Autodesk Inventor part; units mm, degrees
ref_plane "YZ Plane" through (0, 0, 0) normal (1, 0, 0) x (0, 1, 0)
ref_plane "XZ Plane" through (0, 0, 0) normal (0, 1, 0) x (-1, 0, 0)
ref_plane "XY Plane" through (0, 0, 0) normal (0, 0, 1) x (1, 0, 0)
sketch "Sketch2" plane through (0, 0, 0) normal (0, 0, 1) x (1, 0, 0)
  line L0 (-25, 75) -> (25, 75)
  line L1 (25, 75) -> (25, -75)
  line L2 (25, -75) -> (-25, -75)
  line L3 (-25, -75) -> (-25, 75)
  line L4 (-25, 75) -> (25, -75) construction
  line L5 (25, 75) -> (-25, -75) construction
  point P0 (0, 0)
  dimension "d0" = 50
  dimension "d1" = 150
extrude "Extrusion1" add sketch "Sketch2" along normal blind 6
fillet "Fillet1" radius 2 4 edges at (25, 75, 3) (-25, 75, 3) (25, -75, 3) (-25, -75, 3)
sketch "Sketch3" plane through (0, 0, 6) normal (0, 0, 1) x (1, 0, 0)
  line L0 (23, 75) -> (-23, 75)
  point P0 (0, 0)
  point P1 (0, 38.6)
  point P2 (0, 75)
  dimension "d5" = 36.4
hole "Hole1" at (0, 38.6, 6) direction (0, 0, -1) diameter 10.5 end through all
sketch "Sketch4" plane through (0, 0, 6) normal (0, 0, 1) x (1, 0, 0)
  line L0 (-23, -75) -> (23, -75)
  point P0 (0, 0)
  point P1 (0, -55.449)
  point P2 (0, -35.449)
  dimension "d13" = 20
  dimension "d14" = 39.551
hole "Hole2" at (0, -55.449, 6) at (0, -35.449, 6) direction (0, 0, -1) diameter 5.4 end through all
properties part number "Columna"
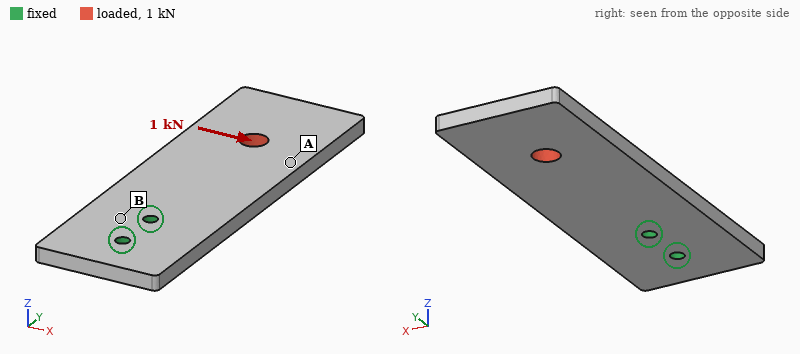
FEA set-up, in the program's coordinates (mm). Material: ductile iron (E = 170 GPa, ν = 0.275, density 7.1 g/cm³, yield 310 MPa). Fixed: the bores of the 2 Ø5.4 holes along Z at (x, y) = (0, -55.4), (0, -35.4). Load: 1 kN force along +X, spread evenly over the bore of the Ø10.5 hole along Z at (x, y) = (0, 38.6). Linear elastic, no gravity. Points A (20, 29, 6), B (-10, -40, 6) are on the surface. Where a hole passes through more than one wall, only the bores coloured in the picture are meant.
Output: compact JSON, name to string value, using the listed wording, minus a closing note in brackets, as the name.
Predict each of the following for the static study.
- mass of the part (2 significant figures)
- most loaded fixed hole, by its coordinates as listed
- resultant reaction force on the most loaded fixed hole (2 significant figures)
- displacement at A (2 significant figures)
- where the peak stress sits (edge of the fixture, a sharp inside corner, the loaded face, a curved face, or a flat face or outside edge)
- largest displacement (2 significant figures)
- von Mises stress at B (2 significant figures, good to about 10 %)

{"mass of the part": "310 g", "most loaded fixed hole, by its coordinates as listed": "(0, -35.4)", "resultant reaction force on the most loaded fixed hole": "3.9 kN", "displacement at A": "35 µm", "where the peak stress sits": "edge of the fixture", "largest displacement": "60 µm", "von Mises stress at B": "27 MPa"}
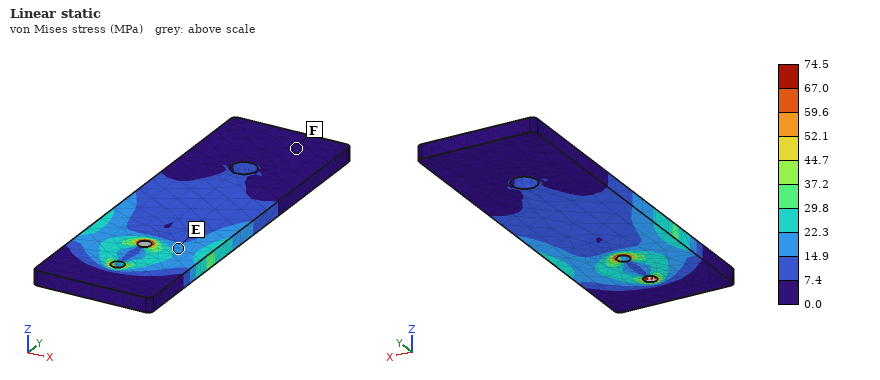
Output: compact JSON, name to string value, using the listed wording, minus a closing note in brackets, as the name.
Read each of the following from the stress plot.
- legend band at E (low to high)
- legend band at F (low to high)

{"legend band at E": "14.9 to 22.3 MPa", "legend band at F": "0.0 to 7.4 MPa"}
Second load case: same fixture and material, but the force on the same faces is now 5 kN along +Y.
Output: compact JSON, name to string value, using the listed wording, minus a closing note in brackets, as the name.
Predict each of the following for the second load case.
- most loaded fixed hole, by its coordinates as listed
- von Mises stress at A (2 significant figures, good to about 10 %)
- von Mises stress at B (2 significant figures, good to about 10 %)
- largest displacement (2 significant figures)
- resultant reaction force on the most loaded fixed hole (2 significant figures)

{"most loaded fixed hole, by its coordinates as listed": "(0, -35.4)", "von Mises stress at A": "11 MPa", "von Mises stress at B": "14 MPa", "largest displacement": "11 µm", "resultant reaction force on the most loaded fixed hole": "3.5 kN"}
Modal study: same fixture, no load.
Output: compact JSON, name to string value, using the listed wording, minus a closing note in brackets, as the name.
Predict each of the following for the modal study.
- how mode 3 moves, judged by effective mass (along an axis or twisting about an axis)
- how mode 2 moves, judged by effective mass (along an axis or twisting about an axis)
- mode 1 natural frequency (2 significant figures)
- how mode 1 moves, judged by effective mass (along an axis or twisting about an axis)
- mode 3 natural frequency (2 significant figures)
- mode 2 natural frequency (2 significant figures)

{"how mode 3 moves, judged by effective mass": "along X", "how mode 2 moves, judged by effective mass": "twisting about Y", "mode 1 natural frequency": "380 Hz", "how mode 1 moves, judged by effective mass": "along Z", "mode 3 natural frequency": "1900 Hz", "mode 2 natural frequency": "1500 Hz"}
